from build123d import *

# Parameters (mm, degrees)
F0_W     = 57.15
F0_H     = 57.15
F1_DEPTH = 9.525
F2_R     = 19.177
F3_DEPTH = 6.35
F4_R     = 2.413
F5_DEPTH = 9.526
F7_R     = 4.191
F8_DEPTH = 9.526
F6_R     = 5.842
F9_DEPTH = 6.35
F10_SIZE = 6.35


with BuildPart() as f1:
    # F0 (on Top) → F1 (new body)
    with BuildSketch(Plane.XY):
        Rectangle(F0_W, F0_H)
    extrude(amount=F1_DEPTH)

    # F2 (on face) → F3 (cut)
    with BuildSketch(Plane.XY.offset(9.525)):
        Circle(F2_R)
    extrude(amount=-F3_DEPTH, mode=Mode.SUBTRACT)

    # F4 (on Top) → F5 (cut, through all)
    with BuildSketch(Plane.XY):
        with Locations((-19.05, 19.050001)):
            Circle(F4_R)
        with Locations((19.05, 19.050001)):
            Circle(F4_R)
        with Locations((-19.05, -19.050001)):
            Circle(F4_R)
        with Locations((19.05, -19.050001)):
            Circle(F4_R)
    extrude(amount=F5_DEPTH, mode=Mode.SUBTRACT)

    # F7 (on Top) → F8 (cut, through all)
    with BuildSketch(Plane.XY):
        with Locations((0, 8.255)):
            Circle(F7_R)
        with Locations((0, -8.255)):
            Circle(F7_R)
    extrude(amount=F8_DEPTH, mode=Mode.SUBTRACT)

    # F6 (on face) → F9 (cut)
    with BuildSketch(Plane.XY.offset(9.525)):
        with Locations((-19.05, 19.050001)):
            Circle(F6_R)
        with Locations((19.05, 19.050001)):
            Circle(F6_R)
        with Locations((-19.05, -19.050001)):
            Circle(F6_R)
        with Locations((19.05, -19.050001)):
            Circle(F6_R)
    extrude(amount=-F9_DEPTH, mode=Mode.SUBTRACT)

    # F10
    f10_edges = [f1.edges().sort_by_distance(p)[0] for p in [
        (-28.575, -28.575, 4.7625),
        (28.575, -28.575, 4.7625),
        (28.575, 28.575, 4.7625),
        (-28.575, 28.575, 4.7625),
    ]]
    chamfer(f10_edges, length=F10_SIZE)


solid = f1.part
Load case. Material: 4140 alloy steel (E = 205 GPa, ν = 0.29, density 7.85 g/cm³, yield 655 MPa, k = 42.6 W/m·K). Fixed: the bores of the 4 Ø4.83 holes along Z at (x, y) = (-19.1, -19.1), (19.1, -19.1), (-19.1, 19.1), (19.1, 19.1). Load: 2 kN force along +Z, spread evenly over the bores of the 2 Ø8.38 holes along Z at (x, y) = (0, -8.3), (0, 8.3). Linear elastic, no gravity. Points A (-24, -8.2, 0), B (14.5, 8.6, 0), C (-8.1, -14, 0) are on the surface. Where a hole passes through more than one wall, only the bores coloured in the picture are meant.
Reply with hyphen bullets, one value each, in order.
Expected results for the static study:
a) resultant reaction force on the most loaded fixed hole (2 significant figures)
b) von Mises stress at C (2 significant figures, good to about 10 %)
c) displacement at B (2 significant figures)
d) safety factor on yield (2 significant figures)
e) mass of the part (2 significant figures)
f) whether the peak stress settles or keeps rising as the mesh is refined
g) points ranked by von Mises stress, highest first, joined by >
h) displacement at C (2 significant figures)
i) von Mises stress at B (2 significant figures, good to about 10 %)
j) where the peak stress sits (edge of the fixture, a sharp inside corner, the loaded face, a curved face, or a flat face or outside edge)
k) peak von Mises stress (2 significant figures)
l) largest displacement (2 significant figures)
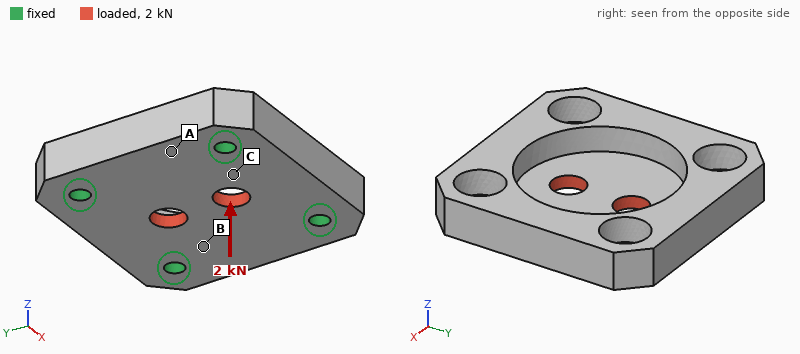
- 620 N
- 65 MPa
- 6.0 µm
- 3.0
- 150 g
- settles
- C > B > A
- 8.4 µm
- 51 MPa
- the loaded face
- 220 MPa
- 30 µm
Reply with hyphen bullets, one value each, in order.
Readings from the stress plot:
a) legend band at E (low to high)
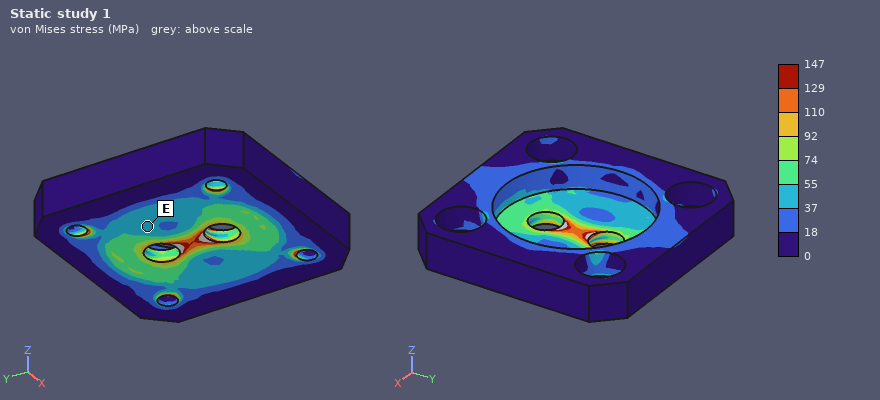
- 37 to 55 MPa
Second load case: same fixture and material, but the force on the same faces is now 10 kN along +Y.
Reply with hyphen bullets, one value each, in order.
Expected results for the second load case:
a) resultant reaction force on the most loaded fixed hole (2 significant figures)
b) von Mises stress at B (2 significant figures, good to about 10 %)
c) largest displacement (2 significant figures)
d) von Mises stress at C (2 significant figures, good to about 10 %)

- 2.6 kN
- 40 MPa
- 9.4 µm
- 50 MPa
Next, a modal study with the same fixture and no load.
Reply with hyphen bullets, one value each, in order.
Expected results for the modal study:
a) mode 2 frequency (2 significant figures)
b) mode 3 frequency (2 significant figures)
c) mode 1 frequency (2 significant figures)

- 13 kHz
- 16 kHz
- 13 kHz
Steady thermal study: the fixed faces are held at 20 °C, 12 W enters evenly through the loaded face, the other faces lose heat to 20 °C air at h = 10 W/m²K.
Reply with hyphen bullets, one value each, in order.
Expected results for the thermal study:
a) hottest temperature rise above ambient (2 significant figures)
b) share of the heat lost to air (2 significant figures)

- 23 K
- 4.7 %
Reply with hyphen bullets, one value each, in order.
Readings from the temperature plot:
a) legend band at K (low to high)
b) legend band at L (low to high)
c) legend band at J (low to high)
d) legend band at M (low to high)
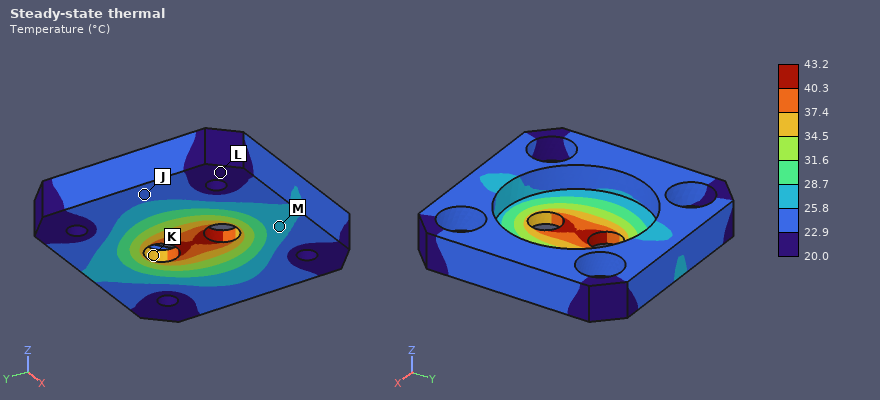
- 34.5 to 37.4 °C
- 20.0 to 22.9 °C
- 22.9 to 25.8 °C
- 25.8 to 28.7 °C
